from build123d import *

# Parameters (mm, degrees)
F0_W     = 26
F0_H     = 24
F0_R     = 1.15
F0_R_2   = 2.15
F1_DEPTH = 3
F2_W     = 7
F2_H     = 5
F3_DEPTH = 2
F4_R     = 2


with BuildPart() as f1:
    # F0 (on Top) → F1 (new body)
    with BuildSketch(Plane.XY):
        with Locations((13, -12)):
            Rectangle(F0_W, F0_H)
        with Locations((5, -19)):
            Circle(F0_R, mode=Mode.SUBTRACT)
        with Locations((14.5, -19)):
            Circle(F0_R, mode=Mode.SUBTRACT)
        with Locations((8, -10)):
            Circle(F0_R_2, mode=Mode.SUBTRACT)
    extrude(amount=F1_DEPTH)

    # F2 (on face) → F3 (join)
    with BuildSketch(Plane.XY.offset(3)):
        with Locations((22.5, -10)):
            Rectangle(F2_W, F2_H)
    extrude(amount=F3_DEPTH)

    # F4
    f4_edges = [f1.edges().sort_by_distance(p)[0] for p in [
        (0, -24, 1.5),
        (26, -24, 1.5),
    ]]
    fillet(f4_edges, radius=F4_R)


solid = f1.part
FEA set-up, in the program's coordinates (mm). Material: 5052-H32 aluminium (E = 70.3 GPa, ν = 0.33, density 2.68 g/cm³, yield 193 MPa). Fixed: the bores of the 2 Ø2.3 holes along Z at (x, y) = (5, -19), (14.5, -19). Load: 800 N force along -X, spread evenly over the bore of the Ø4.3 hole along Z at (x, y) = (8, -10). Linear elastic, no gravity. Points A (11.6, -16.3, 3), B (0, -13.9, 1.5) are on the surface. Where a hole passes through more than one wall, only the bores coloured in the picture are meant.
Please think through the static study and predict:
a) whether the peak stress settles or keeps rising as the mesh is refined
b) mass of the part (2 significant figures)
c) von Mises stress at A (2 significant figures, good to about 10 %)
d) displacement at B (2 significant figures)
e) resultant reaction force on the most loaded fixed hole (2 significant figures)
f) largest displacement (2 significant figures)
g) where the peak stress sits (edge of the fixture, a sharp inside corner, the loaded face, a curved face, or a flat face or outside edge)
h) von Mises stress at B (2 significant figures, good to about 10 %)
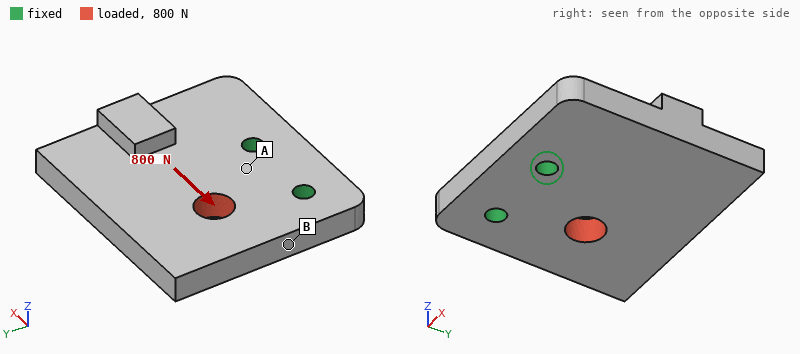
keeps rising
5.0 g
38 MPa
7.4 µm
740 N
18 µm
edge of the fixture
12 MPa
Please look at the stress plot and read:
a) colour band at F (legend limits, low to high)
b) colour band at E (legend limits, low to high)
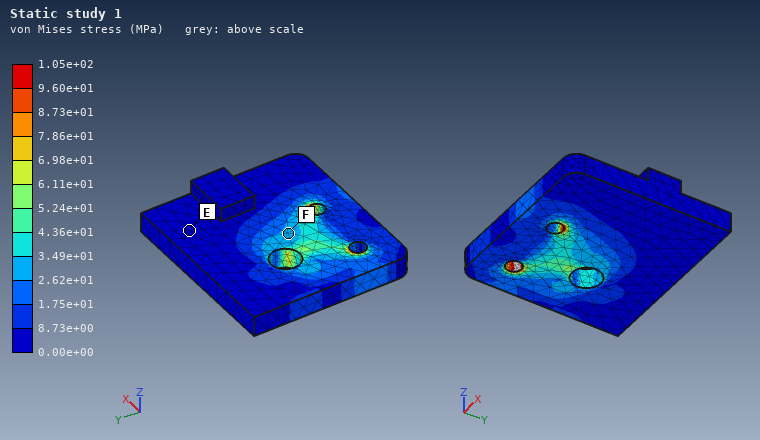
2.62e+01 to 3.49e+01 MPa
0.00e+00 to 8.73e+00 MPa
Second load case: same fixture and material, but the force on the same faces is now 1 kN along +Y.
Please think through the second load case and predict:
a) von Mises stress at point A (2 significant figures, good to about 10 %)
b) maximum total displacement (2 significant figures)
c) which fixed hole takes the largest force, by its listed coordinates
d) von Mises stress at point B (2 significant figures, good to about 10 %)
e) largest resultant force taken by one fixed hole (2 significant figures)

16 MPa
5.2 µm
(5, -19)
8.2 MPa
670 N
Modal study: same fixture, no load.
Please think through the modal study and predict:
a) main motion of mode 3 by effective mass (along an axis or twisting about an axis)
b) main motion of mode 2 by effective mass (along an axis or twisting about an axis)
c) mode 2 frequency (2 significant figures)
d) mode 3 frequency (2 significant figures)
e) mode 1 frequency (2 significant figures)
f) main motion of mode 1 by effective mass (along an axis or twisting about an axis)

along X
twisting about Y
10 kHz
18 kHz
6000 Hz
along Z
